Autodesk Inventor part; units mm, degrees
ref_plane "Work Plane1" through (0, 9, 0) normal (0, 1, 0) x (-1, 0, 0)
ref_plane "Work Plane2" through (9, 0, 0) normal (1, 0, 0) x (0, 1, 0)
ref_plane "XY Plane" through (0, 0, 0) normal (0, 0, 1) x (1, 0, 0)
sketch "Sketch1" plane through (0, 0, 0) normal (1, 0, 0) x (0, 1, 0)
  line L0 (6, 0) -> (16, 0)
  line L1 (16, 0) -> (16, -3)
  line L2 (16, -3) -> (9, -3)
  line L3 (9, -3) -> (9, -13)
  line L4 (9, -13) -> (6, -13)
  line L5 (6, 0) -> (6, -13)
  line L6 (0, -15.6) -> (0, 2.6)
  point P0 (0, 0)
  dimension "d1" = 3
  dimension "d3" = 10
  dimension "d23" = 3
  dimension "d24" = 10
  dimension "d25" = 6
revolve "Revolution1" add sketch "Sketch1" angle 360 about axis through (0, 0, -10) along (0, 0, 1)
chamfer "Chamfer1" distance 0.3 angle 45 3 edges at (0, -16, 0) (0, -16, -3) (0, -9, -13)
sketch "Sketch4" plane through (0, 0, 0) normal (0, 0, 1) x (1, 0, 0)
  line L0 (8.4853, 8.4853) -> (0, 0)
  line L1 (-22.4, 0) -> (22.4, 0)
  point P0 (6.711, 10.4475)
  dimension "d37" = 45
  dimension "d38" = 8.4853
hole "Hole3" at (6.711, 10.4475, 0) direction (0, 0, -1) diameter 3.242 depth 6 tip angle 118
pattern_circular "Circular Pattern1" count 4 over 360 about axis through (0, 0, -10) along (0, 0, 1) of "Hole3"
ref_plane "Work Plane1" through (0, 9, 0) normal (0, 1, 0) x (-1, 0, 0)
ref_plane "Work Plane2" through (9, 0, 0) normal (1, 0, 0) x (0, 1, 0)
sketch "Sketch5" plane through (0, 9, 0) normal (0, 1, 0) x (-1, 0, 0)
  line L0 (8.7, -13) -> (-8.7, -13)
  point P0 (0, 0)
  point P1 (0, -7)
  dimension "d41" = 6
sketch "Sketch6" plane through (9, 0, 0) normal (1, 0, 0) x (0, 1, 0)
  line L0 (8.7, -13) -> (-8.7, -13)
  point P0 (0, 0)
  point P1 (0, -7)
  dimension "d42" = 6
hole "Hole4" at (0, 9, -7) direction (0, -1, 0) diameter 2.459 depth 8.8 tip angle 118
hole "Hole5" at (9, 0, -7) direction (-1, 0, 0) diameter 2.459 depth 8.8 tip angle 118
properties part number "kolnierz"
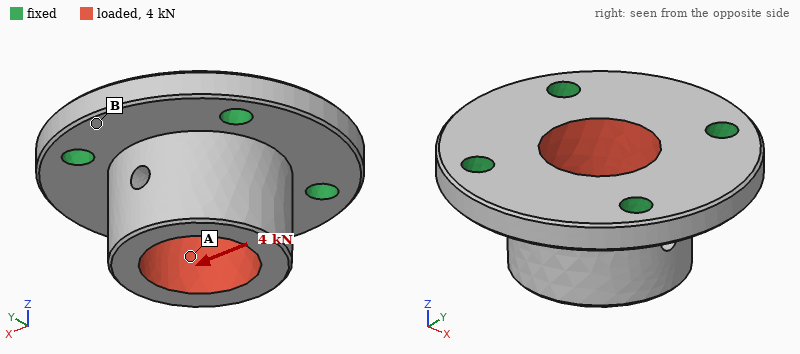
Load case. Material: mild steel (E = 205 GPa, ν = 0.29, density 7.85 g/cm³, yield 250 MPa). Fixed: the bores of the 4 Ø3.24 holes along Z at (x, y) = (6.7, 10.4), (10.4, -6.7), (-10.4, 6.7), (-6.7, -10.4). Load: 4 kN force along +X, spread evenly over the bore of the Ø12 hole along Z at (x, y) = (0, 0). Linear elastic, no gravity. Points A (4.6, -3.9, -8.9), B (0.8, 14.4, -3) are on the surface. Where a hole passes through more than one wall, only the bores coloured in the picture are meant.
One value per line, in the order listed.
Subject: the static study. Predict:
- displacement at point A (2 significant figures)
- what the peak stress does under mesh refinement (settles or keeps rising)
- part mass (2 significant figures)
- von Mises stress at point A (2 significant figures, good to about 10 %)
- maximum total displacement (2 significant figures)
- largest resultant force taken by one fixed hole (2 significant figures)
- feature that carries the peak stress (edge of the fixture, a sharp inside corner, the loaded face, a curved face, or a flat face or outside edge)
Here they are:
5.4 µm
keeps rising
26 g
39 MPa
8.6 µm
1.3 kN
edge of the fixture
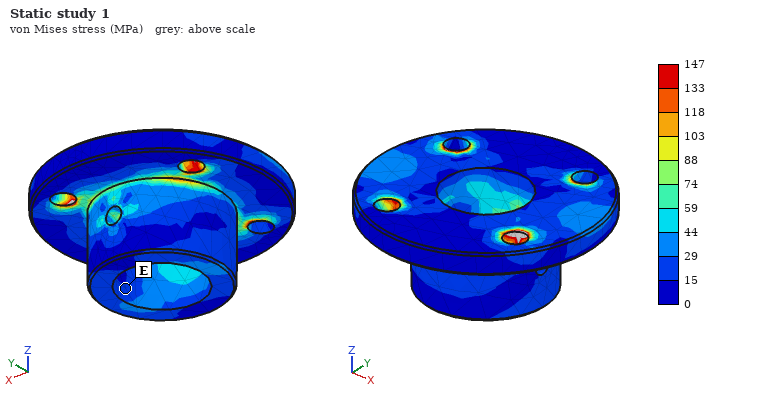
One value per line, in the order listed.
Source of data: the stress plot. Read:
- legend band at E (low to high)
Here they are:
15 to 29 MPa
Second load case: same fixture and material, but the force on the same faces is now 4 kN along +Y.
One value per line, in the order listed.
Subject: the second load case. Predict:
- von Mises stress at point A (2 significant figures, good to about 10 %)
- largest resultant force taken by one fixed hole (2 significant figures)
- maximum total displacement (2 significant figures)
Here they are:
30 MPa
1.3 kN
8.6 µm
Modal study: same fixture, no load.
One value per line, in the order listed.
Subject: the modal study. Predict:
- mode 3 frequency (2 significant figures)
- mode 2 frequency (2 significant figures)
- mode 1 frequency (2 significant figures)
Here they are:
37 kHz
31 kHz
31 kHz
